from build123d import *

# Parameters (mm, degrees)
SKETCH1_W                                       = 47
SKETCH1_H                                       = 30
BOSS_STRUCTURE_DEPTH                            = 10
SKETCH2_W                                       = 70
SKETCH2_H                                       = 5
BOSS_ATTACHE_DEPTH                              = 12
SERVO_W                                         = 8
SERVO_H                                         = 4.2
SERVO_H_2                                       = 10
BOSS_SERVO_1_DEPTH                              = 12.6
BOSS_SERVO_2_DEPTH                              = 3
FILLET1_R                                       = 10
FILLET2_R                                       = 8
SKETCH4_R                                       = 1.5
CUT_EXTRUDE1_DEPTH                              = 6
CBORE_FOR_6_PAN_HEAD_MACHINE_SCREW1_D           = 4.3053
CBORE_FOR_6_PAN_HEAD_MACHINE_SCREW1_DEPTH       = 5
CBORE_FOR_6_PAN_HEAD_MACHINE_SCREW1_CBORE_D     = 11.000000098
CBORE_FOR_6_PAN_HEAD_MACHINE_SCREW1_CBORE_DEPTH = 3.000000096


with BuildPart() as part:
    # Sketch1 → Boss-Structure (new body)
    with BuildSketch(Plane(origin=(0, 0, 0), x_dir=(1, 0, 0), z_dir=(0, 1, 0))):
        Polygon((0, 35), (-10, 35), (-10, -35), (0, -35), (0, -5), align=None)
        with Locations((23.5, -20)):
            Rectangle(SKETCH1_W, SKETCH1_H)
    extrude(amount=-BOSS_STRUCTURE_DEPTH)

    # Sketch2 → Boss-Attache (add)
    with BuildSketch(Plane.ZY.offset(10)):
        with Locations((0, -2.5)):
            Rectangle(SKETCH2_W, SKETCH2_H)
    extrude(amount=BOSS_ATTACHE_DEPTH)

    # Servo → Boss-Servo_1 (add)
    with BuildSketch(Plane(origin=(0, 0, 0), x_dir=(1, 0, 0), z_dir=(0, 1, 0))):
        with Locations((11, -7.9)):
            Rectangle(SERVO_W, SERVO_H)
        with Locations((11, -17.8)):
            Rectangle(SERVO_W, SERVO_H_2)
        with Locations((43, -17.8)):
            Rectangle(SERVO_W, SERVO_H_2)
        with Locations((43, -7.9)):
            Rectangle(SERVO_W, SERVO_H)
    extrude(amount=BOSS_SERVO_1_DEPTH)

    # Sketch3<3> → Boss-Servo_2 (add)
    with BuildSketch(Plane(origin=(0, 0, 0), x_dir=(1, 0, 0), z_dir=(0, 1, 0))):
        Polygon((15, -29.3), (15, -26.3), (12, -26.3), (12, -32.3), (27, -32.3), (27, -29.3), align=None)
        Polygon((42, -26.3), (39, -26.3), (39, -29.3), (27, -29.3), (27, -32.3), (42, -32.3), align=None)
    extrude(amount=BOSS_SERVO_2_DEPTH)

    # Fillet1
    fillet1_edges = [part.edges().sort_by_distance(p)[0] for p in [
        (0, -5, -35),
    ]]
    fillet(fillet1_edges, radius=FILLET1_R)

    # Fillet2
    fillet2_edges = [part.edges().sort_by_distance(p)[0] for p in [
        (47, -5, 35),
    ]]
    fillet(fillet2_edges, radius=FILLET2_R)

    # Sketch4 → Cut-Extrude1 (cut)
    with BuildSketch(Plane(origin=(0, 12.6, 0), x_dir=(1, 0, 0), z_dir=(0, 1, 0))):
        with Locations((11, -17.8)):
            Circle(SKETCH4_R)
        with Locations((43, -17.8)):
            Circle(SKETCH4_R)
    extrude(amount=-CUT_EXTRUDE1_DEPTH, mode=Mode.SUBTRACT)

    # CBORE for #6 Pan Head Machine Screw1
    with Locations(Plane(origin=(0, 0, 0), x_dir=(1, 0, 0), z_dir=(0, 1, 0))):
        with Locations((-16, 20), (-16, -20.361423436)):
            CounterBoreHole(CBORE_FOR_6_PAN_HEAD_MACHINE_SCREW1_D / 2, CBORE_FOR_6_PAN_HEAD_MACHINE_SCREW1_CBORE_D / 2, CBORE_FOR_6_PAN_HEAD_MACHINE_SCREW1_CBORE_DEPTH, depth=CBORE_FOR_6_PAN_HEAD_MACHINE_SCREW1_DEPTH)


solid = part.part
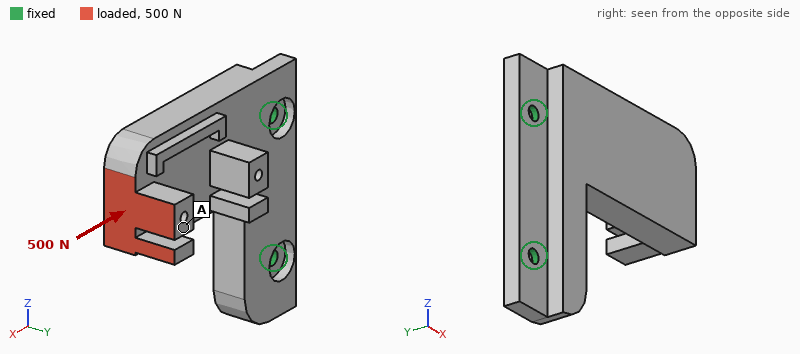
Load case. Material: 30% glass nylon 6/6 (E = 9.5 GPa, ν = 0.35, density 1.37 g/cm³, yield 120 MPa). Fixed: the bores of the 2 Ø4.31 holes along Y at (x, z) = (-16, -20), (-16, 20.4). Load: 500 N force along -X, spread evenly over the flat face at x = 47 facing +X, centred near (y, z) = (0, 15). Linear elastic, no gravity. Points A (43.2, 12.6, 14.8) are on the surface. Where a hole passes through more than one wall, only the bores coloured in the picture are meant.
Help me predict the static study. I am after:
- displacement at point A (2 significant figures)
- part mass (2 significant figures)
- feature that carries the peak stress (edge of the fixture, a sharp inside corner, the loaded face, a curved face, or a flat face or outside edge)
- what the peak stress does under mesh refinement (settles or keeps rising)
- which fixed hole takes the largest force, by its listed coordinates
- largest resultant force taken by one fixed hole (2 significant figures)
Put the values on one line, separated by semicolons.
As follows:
0.89 mm; 38 g; edge of the fixture; keeps rising; (-16, 20.4); 440 N
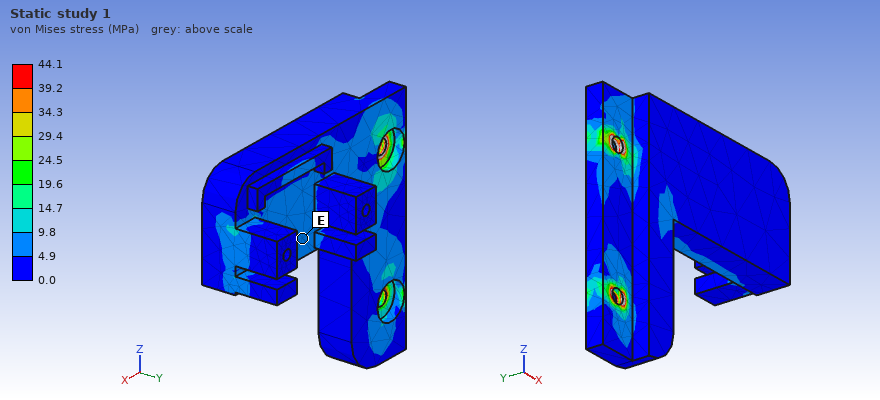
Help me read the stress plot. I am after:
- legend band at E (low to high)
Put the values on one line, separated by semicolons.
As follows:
4.9 to 9.8 MPa
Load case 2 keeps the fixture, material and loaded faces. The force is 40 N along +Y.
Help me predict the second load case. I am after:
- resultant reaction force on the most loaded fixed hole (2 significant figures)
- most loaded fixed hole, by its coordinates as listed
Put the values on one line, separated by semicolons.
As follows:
40 N; (-16, 20.4)
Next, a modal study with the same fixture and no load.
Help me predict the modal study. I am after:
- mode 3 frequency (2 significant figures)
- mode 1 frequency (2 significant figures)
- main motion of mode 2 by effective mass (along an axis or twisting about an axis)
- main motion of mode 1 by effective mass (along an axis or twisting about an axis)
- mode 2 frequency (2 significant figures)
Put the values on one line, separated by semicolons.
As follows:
2400 Hz; 310 Hz; along Z; along Y; 1600 Hz
